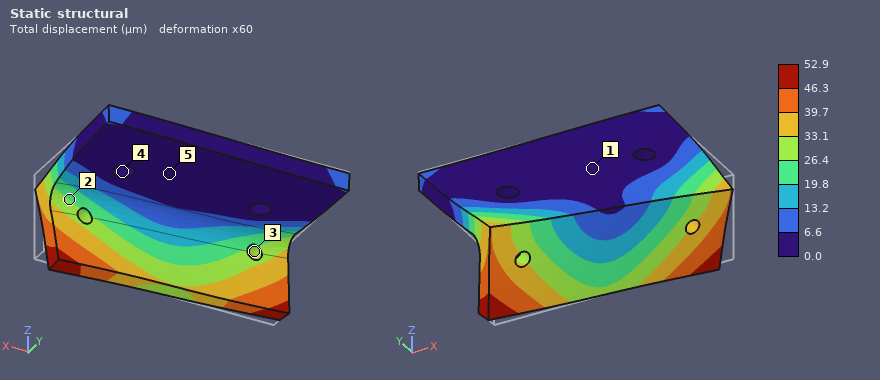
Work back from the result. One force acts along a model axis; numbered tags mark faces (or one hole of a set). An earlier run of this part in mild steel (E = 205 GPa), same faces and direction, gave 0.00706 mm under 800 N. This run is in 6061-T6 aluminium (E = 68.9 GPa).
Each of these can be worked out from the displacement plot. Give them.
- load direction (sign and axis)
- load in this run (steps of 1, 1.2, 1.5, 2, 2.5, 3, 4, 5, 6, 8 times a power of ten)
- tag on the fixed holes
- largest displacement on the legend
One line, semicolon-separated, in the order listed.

-X; 2 kN; 4; 52.9 µm
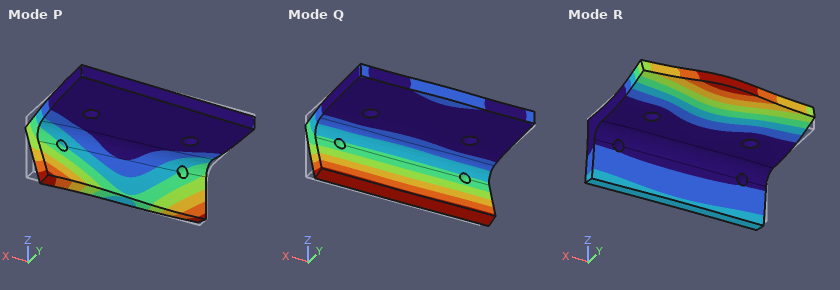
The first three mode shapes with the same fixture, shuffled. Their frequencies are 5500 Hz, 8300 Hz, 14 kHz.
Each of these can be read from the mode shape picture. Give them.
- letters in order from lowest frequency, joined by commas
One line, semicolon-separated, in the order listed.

Q, P, R
